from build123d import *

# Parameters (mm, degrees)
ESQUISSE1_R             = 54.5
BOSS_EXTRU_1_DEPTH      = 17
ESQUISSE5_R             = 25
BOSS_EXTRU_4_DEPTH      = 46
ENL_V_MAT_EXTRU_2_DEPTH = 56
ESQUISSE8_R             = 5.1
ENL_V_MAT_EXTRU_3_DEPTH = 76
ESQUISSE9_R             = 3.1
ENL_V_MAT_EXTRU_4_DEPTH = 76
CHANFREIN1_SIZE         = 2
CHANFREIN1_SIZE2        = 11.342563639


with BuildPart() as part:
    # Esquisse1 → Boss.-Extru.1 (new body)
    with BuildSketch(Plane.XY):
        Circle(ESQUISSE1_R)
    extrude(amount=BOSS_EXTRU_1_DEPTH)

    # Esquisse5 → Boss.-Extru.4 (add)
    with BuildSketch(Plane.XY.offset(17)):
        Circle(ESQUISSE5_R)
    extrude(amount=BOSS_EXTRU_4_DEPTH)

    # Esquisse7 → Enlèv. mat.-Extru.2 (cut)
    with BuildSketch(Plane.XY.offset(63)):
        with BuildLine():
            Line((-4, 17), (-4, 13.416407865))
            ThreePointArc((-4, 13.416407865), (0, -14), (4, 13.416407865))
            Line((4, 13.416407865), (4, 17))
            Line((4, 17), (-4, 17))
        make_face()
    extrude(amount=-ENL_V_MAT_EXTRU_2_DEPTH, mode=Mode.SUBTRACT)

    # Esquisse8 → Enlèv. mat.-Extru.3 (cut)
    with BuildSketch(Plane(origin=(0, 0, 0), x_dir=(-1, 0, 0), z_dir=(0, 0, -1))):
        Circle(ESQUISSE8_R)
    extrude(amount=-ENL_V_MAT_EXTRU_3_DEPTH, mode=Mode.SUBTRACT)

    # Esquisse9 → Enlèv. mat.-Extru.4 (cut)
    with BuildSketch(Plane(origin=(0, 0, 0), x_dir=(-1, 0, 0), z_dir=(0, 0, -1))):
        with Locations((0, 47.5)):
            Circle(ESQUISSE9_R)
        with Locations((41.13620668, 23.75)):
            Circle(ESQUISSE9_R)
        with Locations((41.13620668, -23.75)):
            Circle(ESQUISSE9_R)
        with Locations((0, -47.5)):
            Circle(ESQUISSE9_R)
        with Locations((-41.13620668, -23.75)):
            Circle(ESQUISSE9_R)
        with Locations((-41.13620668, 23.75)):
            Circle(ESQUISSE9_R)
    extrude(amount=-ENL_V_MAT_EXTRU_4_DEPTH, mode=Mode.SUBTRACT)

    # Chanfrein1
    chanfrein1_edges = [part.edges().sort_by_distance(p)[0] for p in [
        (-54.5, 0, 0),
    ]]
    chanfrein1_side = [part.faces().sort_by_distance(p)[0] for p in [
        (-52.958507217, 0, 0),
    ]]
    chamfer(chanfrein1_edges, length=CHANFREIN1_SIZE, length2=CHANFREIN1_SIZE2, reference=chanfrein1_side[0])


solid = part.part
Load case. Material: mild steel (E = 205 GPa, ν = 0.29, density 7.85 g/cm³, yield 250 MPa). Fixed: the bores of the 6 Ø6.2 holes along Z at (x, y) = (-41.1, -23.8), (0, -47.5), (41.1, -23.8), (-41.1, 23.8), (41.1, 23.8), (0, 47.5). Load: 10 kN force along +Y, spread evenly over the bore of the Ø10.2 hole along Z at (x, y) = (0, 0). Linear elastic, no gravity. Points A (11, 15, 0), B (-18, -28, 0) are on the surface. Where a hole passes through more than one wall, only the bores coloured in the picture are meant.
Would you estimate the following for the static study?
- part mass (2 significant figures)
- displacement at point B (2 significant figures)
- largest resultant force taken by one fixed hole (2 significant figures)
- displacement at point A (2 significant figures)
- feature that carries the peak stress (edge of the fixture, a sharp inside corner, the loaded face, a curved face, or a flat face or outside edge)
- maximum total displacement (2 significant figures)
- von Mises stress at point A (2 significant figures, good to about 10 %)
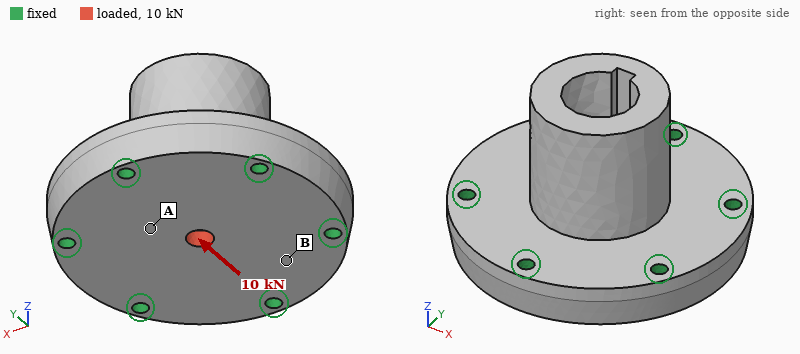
1.6 kg
0.72 µm
2.6 kN
1.4 µm
the loaded face
3.6 µm
14 MPa
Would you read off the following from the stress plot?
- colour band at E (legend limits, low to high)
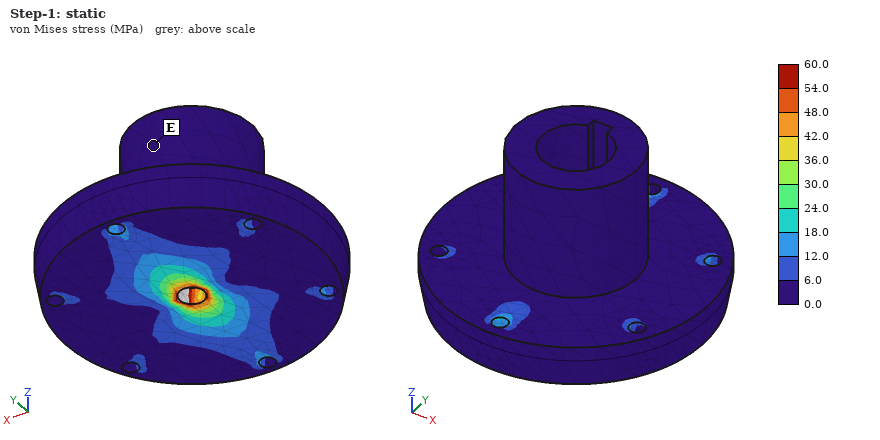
0.0 to 6.0 MPa
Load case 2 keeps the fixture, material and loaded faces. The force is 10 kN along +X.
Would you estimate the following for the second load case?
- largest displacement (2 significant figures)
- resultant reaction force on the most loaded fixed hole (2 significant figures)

3.6 µm
2.3 kN
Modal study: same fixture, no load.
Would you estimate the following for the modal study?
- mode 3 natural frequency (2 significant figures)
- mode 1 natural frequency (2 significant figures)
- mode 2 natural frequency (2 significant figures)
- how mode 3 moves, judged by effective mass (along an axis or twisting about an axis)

9300 Hz
7000 Hz
7000 Hz
along Z
